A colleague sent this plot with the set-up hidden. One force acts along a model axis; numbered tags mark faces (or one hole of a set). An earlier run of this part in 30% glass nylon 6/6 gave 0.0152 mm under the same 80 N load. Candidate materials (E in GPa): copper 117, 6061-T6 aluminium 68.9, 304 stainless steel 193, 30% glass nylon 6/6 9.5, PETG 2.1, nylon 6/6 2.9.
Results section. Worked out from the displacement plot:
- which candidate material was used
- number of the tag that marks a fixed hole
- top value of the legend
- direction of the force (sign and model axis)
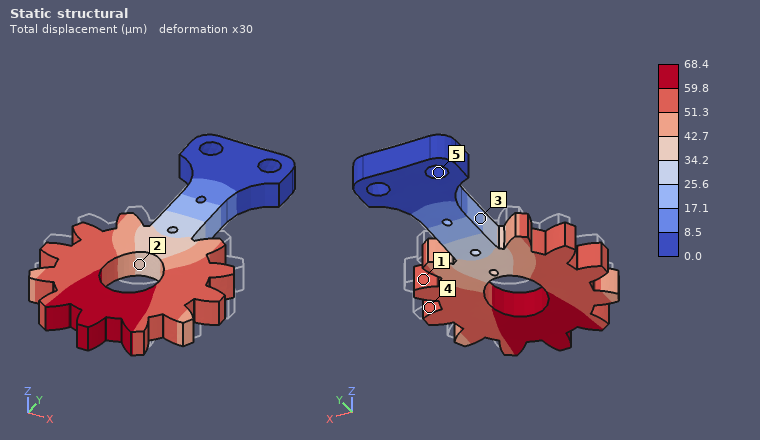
PETG
5
68.4 µm
-Y
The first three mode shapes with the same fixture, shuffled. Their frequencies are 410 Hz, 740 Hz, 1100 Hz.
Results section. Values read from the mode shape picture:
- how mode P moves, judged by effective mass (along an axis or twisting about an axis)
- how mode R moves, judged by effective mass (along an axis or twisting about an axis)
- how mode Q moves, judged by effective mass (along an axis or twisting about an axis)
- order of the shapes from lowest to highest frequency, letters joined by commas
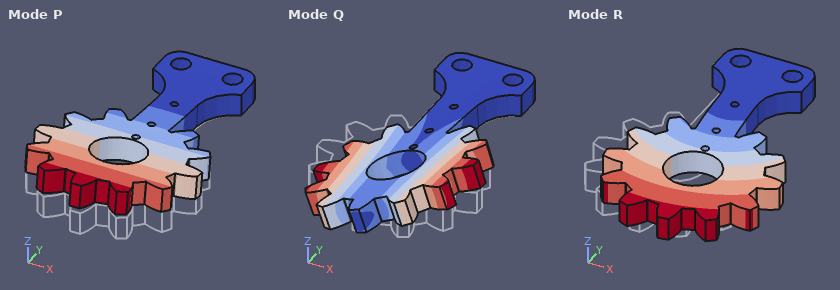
along Z
along X
twisting about Y
P, R, Q
